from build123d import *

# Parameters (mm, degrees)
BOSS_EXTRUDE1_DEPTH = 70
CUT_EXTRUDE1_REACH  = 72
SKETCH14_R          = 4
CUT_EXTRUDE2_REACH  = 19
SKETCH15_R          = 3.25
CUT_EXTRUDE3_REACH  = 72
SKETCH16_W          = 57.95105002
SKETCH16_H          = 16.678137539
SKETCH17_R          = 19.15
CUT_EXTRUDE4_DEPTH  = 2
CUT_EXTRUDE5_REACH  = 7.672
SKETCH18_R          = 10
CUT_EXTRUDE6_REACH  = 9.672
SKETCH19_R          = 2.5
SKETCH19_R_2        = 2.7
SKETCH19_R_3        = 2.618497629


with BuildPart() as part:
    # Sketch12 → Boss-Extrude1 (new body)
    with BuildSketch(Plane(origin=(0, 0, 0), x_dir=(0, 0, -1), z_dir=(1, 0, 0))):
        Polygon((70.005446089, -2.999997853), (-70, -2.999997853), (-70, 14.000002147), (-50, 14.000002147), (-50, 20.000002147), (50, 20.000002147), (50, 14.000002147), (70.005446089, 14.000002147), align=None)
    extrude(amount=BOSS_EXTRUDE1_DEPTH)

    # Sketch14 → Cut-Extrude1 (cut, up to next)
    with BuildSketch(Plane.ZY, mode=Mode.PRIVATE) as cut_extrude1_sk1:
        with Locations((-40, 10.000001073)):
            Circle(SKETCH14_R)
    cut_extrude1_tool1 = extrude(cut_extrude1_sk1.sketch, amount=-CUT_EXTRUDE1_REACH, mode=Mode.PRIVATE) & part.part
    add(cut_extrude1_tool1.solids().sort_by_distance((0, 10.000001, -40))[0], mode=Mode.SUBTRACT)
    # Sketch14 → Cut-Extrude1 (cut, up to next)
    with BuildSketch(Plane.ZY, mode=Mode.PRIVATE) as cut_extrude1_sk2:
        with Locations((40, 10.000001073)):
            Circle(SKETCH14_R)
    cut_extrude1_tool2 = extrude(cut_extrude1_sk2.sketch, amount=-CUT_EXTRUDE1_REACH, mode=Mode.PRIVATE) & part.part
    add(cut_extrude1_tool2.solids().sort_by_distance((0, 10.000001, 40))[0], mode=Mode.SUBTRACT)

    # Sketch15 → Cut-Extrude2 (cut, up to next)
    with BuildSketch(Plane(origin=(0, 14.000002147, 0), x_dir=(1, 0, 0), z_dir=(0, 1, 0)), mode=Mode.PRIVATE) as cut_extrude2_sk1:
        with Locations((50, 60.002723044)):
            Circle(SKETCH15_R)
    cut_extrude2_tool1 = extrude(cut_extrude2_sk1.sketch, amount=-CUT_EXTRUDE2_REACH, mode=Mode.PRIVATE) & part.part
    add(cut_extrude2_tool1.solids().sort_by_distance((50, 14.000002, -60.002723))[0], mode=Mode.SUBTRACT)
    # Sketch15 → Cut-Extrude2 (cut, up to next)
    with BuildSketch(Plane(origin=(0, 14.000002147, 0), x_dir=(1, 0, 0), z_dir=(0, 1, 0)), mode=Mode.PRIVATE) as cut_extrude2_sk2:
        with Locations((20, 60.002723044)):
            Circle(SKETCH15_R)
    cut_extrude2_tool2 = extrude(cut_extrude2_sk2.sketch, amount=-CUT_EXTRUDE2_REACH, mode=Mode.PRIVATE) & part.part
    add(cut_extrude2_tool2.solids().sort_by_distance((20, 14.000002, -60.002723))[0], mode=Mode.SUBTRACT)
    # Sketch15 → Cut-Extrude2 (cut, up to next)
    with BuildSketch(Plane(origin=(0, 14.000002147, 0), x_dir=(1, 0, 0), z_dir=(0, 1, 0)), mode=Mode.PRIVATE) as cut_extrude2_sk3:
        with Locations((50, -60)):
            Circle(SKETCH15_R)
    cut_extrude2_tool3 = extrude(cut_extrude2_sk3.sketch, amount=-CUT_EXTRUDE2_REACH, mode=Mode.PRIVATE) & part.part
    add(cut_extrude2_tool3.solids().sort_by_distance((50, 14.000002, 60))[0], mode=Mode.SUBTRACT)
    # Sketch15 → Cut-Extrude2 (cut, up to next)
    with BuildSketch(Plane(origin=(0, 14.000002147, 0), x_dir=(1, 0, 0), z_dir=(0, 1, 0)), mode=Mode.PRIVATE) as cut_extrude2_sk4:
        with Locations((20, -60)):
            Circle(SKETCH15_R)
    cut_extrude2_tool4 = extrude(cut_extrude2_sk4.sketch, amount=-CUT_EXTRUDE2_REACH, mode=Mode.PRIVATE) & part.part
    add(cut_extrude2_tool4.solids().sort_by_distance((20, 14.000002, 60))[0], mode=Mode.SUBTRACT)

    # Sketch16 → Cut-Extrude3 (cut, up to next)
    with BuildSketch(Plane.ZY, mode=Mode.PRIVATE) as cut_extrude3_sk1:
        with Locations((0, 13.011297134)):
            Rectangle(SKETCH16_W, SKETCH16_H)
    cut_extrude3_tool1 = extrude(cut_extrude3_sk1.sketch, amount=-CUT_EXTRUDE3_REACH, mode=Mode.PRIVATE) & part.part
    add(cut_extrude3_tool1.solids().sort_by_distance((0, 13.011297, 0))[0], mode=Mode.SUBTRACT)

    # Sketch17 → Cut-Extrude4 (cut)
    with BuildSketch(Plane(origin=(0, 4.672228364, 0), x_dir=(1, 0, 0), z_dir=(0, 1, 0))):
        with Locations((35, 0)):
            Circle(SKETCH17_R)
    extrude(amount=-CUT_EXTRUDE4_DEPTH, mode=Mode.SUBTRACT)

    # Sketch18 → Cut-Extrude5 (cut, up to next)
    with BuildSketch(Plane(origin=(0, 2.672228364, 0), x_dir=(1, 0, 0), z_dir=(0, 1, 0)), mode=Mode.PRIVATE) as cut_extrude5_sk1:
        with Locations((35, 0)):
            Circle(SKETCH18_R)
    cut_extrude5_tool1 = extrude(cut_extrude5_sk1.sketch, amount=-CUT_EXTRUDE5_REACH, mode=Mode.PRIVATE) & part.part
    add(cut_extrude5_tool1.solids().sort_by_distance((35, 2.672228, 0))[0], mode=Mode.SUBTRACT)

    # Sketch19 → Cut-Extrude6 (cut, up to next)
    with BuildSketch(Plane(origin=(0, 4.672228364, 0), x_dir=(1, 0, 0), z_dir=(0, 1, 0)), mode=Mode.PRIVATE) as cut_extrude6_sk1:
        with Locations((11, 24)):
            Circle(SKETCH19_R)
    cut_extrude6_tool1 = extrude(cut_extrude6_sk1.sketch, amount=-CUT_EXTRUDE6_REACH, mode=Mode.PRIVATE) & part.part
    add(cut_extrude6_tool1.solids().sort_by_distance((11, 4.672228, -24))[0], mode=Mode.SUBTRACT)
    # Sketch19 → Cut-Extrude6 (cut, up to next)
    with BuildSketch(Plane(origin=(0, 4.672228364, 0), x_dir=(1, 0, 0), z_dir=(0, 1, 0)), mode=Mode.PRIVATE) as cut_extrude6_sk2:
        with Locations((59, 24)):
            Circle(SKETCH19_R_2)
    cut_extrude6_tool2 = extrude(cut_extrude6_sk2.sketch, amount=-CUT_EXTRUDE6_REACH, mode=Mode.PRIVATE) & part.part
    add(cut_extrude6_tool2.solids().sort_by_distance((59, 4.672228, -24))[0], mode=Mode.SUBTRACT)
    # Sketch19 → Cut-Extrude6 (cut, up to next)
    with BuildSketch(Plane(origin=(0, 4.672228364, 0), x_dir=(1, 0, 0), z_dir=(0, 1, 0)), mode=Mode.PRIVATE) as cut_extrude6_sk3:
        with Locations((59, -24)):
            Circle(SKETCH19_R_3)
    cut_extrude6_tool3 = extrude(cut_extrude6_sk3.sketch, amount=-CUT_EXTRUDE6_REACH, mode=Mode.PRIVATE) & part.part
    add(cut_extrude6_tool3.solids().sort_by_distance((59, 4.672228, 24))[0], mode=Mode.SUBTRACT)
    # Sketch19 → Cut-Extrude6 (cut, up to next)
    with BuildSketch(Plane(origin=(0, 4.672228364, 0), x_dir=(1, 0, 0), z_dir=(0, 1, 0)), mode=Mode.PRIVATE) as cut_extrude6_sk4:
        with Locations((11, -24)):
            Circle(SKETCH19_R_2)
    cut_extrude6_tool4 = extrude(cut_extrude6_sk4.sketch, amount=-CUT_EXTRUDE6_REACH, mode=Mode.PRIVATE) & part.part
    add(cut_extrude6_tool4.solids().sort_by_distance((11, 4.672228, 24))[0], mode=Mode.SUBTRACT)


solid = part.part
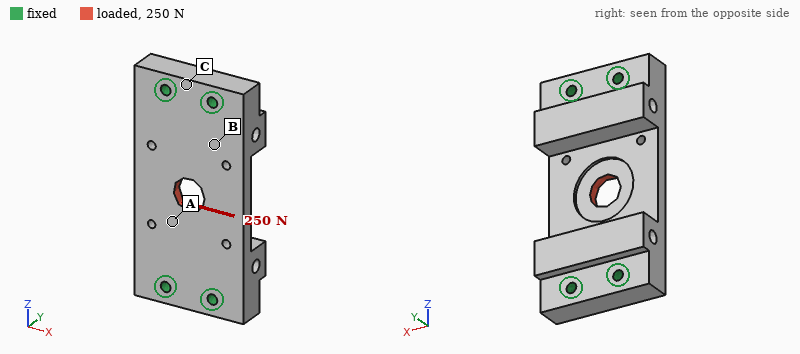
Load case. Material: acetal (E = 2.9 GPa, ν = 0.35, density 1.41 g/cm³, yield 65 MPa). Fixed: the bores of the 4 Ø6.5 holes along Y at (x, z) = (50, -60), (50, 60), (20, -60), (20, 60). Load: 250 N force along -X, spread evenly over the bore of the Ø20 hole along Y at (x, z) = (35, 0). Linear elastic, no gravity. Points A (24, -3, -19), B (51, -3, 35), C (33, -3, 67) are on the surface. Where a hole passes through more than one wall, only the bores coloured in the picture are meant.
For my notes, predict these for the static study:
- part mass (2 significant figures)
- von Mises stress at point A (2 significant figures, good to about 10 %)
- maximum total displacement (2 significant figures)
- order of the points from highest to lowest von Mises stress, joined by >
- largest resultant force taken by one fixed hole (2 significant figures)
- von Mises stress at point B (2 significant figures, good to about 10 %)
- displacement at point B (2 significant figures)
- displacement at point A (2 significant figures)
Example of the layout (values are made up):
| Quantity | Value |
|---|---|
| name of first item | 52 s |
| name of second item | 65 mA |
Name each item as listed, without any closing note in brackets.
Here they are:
| Quantity | Value |
|---|---|
| part mass | 190 g |
| von Mises stress at point A | 0.63 MPa |
| maximum total displacement | 20 µm |
| order of the points from highest to lowest von Mises stress, joined by > | A > B > C |
| largest resultant force taken by one fixed hole | 120 N |
| von Mises stress at point B | 0.40 MPa |
| displacement at point B | 7.4 µm |
| displacement at point A | 13 µm |
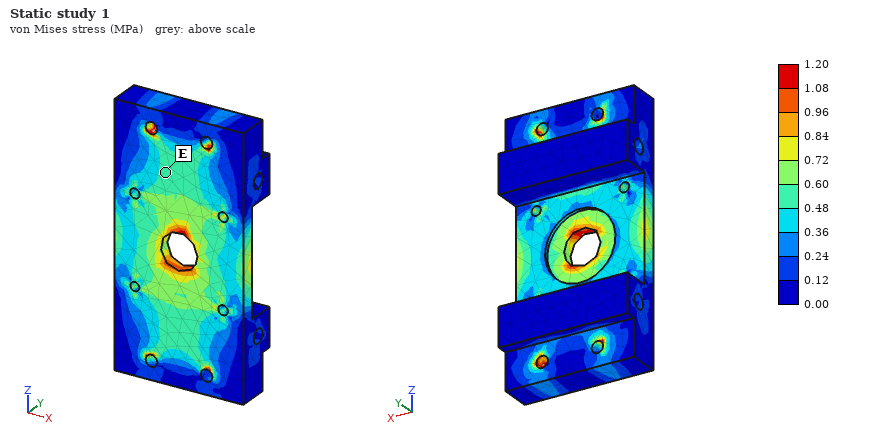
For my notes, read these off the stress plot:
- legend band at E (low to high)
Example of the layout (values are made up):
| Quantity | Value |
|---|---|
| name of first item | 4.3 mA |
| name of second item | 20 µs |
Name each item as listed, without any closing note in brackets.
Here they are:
| Quantity | Value |
|---|---|
| legend band at E | 0.48 to 0.60 MPa |
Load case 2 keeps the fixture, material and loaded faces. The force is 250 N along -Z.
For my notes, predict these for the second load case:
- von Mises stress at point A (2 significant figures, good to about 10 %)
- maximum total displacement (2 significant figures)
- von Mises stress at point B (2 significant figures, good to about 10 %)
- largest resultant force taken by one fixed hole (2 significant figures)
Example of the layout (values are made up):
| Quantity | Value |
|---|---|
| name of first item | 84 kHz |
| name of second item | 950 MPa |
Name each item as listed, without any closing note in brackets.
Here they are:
| Quantity | Value |
|---|---|
| von Mises stress at point A | 0.45 MPa |
| maximum total displacement | 8.0 µm |
| von Mises stress at point B | 0.28 MPa |
| largest resultant force taken by one fixed hole | 63 N |
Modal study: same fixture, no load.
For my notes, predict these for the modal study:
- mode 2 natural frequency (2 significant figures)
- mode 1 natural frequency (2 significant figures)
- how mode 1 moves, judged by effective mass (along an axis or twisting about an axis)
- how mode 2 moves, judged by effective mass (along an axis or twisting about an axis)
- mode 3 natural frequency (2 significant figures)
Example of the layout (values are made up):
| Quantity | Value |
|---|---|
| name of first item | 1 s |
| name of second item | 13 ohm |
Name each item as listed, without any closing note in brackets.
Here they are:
| Quantity | Value |
|---|---|
| mode 2 natural frequency | 2000 Hz |
| mode 1 natural frequency | 1500 Hz |
| how mode 1 moves, judged by effective mass | along Y |
| how mode 2 moves, judged by effective mass | twisting about Z |
| mode 3 natural frequency | 2300 Hz |
